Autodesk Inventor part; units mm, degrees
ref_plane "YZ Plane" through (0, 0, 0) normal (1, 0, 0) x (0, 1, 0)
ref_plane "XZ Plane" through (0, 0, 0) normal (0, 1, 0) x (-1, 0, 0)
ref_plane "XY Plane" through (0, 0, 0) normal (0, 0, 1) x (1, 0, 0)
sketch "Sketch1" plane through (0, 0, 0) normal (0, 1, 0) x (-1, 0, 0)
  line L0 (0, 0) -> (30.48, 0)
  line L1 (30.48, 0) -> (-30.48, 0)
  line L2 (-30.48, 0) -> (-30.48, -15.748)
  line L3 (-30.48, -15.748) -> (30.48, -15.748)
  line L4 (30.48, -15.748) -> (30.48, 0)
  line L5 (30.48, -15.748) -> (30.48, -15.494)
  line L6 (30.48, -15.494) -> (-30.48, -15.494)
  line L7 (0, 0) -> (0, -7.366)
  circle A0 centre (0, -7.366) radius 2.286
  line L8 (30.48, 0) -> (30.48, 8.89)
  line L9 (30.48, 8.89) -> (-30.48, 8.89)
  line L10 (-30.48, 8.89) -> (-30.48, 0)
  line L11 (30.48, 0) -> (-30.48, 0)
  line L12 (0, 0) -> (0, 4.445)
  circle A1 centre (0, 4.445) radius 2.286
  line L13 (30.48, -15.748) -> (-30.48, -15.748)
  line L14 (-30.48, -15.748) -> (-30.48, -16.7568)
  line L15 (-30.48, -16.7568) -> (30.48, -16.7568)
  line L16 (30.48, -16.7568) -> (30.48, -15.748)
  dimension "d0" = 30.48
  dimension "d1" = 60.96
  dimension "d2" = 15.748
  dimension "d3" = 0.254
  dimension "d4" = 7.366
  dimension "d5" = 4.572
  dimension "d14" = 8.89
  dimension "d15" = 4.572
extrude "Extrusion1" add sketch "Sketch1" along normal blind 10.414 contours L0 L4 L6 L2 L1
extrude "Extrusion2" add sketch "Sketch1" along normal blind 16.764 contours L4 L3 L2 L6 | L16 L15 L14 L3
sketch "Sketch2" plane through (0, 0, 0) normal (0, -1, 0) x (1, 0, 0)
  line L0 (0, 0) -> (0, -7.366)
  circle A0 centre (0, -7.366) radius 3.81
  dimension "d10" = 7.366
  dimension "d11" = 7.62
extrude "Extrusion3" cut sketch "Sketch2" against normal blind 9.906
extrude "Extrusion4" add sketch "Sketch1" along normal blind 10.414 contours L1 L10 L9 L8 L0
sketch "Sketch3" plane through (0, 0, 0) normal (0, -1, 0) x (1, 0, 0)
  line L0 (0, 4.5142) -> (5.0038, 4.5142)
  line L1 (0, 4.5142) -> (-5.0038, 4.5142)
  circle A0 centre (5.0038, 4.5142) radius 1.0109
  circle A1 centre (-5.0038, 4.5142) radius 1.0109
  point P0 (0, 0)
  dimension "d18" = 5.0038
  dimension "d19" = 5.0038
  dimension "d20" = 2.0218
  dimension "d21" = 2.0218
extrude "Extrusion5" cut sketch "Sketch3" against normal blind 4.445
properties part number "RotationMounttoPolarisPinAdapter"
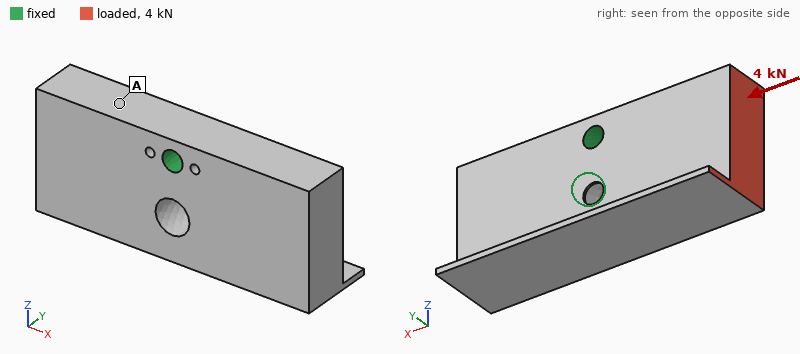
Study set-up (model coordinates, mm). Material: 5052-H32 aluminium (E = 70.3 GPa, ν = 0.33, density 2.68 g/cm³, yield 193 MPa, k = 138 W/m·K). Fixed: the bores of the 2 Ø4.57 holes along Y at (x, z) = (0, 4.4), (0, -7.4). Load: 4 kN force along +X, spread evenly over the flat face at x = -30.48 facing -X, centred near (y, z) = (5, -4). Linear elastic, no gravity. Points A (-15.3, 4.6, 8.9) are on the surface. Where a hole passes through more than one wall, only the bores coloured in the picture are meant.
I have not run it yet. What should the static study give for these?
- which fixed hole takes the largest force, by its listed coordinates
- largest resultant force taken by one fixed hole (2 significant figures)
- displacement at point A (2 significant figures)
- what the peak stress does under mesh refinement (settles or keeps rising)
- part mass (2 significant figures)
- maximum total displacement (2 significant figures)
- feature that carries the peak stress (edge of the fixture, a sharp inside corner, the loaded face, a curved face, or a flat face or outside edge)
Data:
(0, 4.4)
2.3 kN
14 µm
keeps rising
43 g
45 µm
edge of the fixture
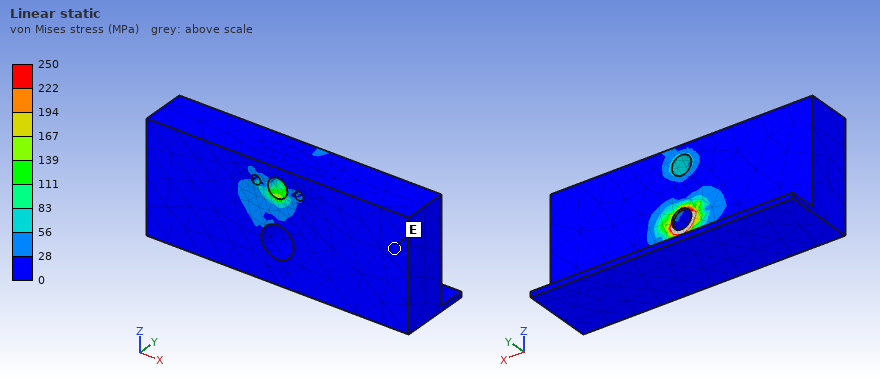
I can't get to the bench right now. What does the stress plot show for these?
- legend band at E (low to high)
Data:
0 to 28 MPa
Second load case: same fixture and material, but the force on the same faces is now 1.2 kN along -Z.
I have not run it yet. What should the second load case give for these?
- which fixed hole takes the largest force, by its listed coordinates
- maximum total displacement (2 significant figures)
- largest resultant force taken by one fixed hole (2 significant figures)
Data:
(0, 4.4)
78 µm
1.9 kN
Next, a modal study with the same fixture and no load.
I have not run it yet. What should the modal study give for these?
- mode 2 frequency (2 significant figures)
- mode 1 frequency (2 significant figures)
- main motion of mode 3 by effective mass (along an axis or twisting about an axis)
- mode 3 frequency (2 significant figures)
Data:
7400 Hz
5300 Hz
along Y
7900 Hz
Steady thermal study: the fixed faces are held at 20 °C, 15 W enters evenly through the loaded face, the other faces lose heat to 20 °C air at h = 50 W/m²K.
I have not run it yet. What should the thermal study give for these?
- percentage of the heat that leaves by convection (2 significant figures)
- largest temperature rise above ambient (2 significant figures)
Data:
8.2 %
14 K
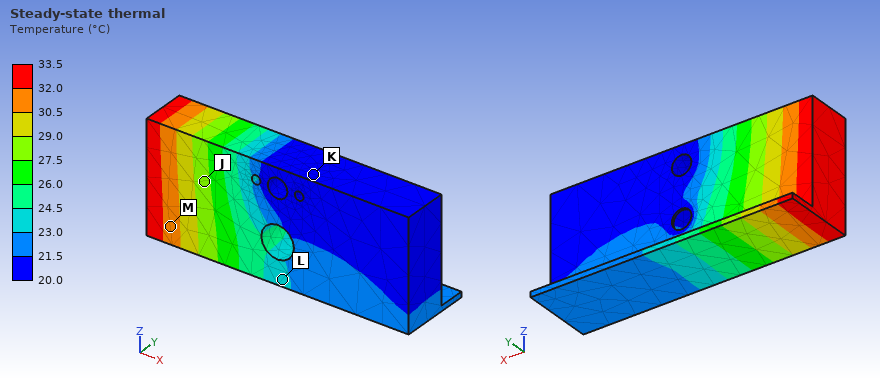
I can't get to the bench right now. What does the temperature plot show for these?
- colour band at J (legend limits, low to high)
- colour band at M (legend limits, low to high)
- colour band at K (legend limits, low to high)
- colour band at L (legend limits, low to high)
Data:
27.5 to 29.0 °C
30.5 to 32.0 °C
20.0 to 21.5 °C
23.0 to 24.5 °C
